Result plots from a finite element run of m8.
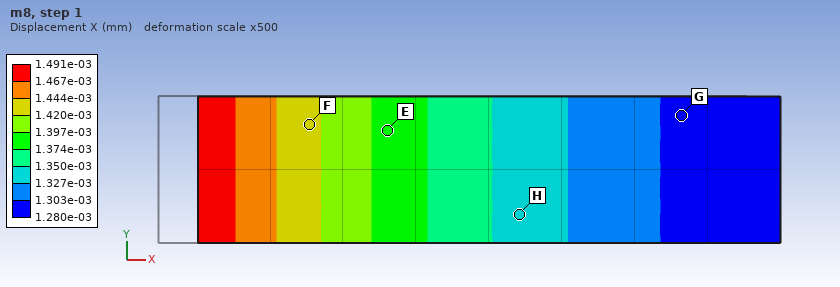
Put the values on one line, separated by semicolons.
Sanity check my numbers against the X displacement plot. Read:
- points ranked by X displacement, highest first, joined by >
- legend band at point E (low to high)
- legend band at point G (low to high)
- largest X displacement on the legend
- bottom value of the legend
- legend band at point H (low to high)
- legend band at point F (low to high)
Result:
F > E > H > G; 1.374e-03 to 1.397e-03 mm; 1.280e-03 to 1.303e-03 mm; 1.491e-03 mm; 1.280e-03 mm; 1.327e-03 to 1.350e-03 mm; 1.420e-03 to 1.444e-03 mm
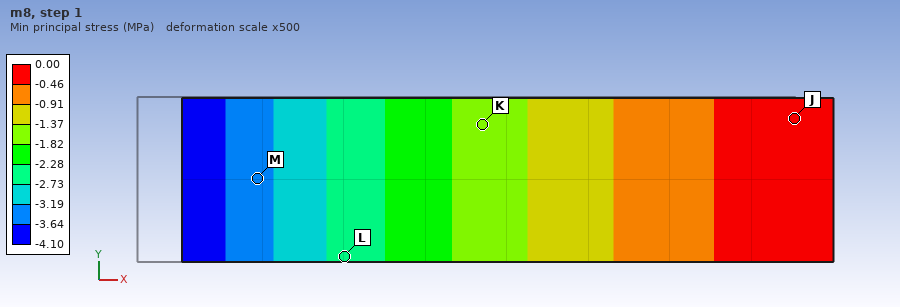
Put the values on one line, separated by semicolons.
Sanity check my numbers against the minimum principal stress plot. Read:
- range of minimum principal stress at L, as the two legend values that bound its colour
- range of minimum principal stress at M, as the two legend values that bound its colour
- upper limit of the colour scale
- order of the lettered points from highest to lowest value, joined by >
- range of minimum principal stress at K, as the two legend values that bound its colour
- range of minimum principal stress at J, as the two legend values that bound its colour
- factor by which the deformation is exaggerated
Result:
-2.73 to -2.28 MPa; -3.64 to -3.19 MPa; 0.00 MPa; J > K > L > M; -1.82 to -1.37 MPa; -0.46 to 0.00 MPa; 500
